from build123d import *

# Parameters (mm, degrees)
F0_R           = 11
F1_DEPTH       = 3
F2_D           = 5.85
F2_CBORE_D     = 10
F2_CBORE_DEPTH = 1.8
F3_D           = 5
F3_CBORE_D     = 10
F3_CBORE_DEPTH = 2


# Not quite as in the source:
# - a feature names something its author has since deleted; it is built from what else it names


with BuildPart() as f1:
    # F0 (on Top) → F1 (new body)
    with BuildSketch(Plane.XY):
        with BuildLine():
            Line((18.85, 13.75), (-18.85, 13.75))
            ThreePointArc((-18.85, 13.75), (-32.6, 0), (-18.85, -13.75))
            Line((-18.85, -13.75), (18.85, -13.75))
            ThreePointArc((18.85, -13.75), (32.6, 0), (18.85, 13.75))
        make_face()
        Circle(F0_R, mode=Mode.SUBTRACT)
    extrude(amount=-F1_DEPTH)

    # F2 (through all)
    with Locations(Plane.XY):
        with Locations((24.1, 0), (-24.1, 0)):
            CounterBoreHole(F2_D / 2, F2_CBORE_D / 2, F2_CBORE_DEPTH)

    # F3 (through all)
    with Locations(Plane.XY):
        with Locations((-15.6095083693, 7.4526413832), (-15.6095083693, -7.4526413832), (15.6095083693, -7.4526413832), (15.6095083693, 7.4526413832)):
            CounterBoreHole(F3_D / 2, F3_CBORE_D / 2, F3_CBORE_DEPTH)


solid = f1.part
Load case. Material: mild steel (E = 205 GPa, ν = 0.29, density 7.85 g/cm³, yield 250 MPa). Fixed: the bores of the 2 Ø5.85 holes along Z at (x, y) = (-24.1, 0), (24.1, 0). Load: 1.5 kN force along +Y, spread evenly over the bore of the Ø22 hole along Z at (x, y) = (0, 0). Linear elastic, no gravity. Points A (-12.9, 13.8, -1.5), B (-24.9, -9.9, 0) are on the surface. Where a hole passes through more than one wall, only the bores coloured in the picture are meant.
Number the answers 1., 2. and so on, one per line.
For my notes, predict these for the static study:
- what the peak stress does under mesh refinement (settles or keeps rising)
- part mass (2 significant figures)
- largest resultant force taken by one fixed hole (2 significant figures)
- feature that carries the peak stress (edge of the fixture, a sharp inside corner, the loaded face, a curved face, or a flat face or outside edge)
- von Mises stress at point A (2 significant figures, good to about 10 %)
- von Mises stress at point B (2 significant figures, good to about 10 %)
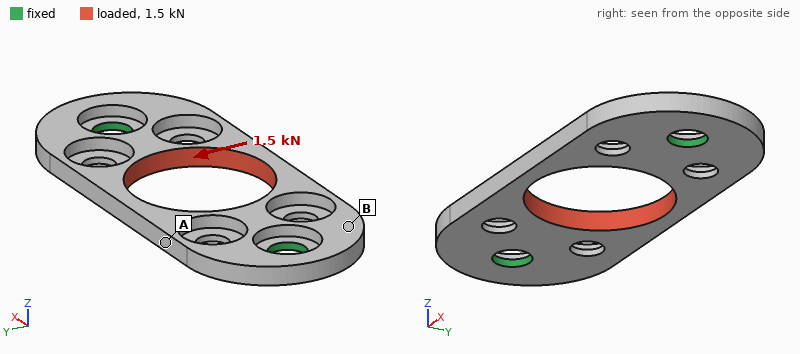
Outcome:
1. keeps rising
2. 21 g
3. 750 N
4. edge of the fixture
5. 46 MPa
6. 13 MPa
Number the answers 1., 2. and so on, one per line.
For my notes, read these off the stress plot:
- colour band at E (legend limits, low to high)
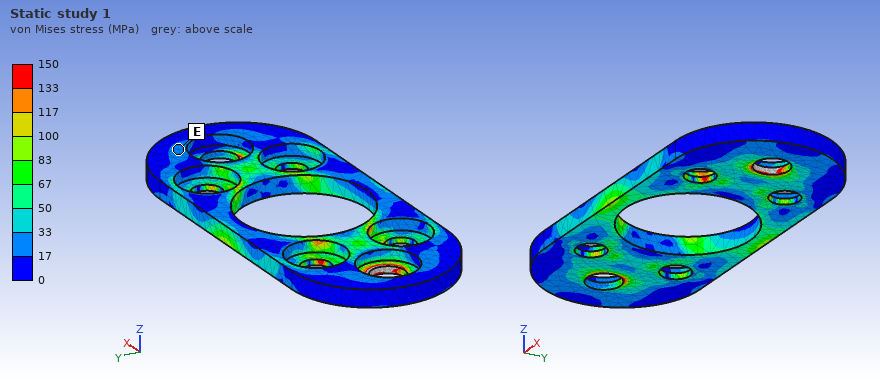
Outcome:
1. 17 to 33 MPa
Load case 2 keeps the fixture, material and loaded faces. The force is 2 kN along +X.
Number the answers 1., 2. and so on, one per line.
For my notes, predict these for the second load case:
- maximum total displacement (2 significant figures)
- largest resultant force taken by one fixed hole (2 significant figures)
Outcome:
1. 6.5 µm
2. 1.0 kN
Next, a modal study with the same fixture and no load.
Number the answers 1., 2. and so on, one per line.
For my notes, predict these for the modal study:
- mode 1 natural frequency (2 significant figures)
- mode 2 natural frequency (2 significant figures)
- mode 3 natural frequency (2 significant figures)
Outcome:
1. 5200 Hz
2. 5200 Hz
3. 9200 Hz
